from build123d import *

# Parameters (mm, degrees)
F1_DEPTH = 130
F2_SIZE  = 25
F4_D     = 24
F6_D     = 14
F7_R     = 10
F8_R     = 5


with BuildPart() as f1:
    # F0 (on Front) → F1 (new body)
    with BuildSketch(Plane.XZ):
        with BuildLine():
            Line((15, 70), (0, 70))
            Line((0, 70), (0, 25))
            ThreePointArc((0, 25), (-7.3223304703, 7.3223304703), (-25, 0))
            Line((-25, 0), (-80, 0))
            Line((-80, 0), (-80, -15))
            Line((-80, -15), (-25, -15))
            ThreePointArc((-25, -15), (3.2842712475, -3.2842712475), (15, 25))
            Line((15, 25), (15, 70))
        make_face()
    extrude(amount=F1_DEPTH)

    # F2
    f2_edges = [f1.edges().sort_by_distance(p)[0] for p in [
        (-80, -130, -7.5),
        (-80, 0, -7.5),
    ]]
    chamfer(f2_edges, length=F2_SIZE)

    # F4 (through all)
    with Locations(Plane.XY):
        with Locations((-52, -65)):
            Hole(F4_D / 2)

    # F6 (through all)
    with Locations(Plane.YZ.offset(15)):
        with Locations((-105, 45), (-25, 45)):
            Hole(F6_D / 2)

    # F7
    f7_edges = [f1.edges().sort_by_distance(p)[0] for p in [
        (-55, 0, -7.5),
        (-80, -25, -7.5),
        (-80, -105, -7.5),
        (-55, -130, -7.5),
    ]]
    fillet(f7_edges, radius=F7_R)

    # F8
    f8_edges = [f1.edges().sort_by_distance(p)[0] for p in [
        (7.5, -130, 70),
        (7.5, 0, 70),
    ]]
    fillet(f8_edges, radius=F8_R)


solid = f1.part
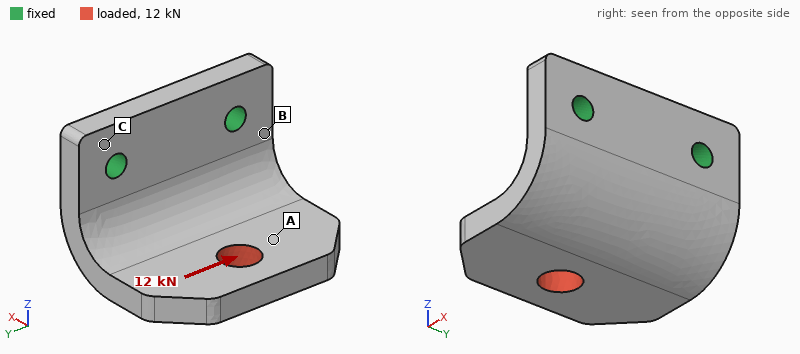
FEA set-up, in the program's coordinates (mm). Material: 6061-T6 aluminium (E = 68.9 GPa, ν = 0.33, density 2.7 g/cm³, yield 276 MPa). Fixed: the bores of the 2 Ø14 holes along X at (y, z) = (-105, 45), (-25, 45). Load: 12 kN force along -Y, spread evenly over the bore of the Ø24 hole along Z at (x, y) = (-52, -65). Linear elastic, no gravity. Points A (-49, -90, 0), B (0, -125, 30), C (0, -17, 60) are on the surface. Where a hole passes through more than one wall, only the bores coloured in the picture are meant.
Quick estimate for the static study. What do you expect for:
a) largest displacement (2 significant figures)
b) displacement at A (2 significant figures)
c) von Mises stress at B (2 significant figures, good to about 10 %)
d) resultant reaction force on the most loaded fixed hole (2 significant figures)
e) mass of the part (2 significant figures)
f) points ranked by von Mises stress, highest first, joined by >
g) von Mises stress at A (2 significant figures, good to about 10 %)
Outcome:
0.31 mm
0.20 mm
51 MPa
12 kN
740 g
B > A > C
27 MPa
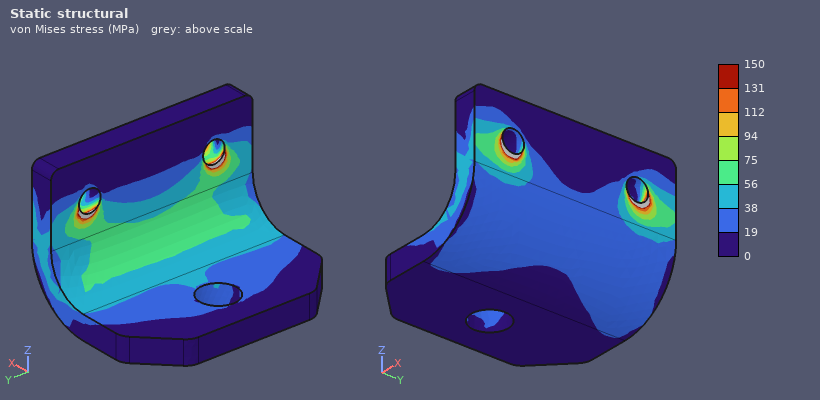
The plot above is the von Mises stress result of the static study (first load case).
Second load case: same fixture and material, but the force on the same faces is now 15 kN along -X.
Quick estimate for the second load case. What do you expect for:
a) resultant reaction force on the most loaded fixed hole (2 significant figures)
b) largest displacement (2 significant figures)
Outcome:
7.5 kN
0.83 mm
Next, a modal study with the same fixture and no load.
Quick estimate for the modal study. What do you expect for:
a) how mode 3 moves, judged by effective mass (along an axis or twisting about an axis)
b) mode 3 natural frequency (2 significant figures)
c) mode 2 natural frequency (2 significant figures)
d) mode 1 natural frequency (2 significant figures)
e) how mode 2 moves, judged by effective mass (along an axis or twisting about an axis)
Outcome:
along X
3200 Hz
1800 Hz
980 Hz
along Y
